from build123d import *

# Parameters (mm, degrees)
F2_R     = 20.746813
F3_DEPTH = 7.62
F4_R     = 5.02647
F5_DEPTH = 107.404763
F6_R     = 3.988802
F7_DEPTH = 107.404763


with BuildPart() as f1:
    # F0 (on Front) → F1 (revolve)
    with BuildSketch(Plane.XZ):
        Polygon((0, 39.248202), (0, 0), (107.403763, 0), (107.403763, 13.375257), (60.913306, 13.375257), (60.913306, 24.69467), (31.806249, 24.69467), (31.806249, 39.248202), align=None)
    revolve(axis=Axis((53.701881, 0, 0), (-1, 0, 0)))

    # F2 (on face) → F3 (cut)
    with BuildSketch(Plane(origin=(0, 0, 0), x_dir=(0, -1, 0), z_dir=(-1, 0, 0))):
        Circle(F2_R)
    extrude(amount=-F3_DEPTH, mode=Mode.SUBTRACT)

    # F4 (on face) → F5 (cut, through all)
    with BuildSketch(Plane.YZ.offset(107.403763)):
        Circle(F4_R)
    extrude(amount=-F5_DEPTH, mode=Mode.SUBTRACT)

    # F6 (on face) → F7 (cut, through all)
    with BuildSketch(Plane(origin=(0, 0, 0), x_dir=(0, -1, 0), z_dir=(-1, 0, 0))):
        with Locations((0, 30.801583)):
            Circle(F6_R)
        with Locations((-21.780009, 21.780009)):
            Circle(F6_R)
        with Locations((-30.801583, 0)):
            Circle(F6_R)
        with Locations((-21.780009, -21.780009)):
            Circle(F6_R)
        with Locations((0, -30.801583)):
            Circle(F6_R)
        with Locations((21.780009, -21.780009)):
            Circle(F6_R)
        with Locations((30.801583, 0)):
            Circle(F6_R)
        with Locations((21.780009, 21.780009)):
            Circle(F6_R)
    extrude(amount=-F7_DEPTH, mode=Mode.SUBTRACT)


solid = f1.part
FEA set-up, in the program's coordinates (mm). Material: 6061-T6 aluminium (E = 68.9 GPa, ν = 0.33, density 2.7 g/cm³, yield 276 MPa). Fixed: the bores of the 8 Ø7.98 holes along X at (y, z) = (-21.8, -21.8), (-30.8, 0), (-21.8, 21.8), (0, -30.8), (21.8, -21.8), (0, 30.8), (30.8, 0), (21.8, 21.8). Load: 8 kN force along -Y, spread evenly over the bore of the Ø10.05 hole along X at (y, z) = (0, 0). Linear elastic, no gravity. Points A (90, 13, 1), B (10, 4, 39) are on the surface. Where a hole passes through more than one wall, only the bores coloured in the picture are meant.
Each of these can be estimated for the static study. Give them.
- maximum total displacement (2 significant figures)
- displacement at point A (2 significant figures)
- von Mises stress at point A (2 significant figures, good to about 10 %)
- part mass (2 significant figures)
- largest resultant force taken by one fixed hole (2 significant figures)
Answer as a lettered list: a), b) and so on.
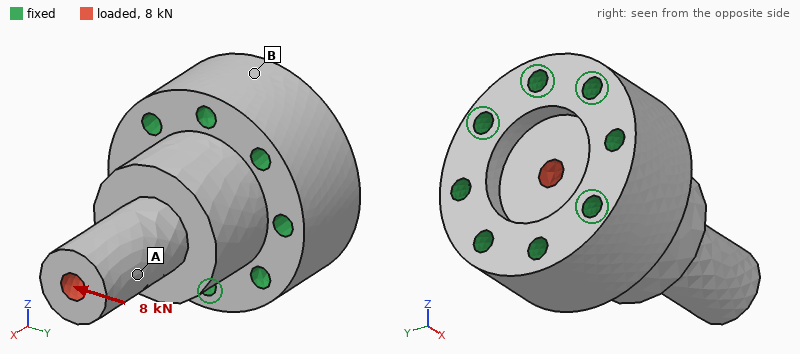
a) 73 µm
b) 50 µm
c) 6.7 MPa
d) 550 g
e) 3.2 kN
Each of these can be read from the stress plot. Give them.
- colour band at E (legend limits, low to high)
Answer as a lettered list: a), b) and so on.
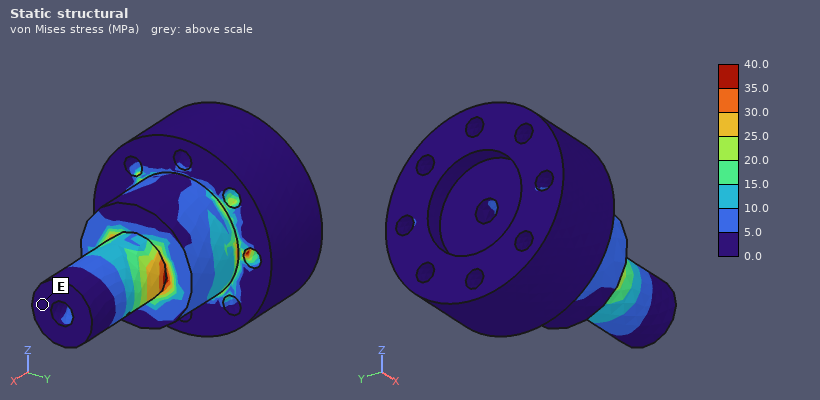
a) 0.0 to 5.0 MPa
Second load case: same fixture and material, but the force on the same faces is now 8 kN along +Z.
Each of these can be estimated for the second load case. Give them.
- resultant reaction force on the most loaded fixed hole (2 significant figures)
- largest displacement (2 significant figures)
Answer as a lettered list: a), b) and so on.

a) 3.2 kN
b) 73 µm
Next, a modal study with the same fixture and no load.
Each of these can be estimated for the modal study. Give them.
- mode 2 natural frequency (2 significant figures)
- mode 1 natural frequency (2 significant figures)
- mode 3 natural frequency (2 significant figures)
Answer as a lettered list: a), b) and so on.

a) 5600 Hz
b) 5600 Hz
c) 14 kHz
